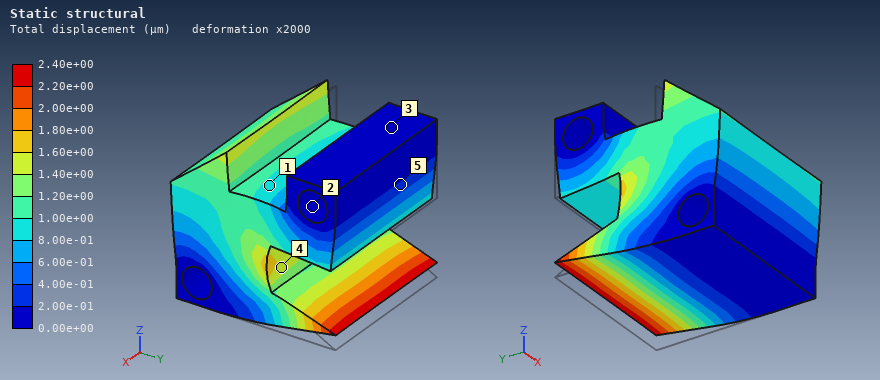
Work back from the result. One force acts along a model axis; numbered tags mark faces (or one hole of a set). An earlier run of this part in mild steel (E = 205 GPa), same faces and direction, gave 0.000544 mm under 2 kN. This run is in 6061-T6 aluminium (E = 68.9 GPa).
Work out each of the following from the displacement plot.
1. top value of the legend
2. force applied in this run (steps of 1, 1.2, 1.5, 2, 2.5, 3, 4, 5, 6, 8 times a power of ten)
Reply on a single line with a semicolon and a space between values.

2.40e+00 µm; 3 kN
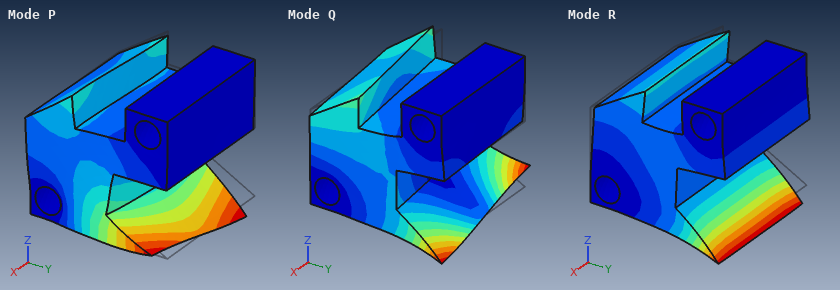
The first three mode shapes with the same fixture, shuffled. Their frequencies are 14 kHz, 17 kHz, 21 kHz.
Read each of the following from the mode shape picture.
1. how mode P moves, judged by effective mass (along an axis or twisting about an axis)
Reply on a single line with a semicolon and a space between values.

along X
